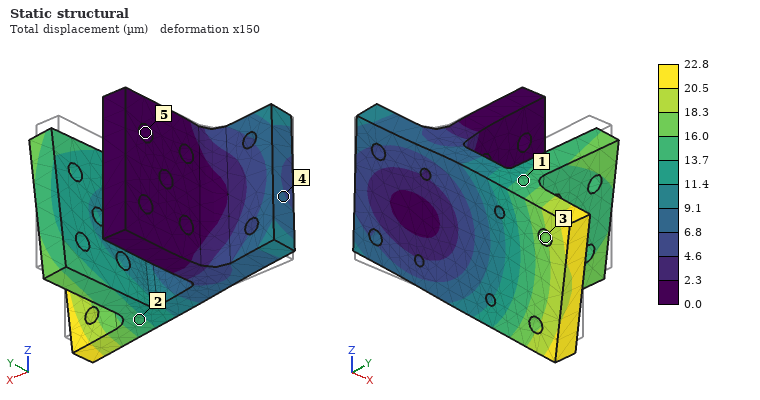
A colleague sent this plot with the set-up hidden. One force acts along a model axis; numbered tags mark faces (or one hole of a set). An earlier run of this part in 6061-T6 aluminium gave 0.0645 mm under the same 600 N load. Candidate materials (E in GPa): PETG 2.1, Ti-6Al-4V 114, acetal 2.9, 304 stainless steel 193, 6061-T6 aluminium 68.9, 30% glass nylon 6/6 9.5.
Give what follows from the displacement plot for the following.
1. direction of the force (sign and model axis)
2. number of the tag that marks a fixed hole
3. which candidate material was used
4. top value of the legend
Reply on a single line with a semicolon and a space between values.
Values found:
-Z; 5; 304 stainless steel; 22.8 µm
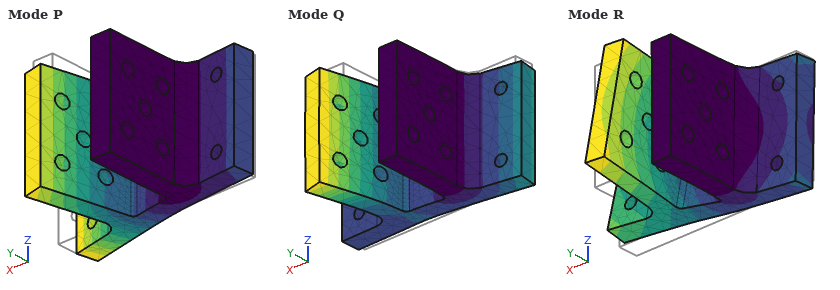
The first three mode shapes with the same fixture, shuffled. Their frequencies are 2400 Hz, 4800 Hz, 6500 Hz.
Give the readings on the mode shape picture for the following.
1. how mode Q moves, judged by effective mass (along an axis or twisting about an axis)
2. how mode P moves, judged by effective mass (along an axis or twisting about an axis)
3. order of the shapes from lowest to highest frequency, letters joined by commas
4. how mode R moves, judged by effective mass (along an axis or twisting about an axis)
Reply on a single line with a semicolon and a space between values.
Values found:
along X; along Y; P, R, Q; along Z
